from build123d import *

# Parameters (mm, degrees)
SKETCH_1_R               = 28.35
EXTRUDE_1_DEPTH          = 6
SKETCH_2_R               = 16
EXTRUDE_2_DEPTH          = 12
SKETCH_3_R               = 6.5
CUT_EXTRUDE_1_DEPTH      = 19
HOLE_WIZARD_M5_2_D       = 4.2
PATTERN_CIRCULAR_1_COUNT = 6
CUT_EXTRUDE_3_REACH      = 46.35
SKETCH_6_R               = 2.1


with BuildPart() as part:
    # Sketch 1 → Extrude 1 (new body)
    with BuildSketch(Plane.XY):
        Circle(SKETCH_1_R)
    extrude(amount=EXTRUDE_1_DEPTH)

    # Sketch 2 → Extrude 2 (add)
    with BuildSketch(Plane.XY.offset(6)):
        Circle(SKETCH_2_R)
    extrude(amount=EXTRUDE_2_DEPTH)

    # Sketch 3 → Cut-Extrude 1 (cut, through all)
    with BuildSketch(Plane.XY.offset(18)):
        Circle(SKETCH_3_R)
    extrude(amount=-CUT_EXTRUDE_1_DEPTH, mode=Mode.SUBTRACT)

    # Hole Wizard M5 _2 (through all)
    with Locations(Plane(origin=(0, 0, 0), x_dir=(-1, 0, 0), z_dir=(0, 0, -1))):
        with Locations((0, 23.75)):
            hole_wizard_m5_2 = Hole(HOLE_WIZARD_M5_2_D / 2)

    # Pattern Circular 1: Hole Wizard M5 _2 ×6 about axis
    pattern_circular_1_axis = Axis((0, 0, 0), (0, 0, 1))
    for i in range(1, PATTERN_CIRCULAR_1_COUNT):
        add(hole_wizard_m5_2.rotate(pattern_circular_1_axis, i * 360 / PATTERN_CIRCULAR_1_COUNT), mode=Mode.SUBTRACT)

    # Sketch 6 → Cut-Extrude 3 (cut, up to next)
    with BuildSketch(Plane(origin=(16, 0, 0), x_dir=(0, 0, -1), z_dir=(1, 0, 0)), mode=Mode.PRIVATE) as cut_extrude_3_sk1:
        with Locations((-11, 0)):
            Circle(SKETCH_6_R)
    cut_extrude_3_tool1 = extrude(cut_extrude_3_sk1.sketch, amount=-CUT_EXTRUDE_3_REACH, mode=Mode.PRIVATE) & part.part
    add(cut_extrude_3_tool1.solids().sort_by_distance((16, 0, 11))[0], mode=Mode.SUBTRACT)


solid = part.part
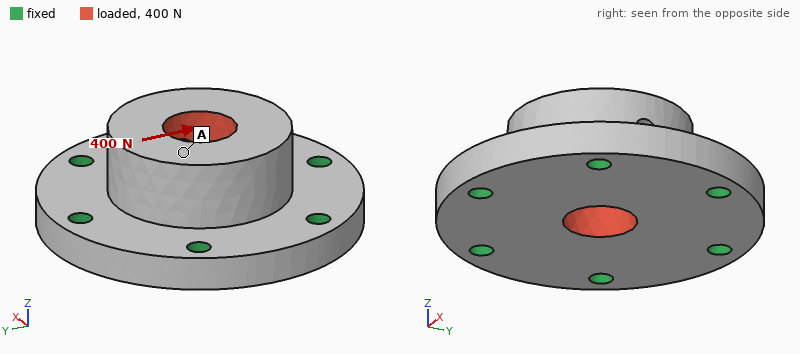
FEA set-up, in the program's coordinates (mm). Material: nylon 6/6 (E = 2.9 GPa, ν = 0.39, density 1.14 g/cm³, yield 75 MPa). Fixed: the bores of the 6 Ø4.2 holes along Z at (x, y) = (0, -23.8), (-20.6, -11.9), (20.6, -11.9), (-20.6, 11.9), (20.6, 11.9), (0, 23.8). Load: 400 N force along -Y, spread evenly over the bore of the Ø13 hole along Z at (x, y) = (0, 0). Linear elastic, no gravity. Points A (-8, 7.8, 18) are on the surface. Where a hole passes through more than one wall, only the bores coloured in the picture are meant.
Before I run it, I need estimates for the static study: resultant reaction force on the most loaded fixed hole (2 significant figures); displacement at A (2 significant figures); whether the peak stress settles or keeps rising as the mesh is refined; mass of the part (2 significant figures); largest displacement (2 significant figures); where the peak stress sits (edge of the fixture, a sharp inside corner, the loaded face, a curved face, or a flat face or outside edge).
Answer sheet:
110 N
13 µm
keeps rising
25 g
15 µm
edge of the fixture
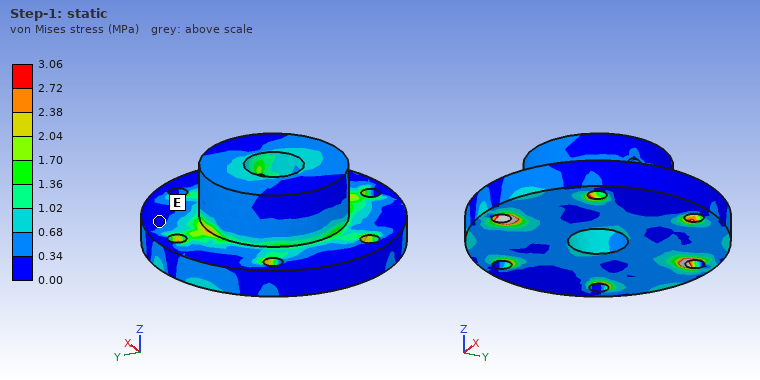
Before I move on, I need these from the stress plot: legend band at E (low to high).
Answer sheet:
0.00 to 0.34 MPa
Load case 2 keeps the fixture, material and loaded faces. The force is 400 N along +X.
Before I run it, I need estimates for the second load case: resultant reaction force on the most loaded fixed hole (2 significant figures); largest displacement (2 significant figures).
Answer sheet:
94 N
15 µm
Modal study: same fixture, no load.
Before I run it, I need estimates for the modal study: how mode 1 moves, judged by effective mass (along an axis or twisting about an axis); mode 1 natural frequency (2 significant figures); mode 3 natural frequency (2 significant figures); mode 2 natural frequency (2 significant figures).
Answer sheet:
along Z
6500 Hz
7600 Hz
7600 Hz
